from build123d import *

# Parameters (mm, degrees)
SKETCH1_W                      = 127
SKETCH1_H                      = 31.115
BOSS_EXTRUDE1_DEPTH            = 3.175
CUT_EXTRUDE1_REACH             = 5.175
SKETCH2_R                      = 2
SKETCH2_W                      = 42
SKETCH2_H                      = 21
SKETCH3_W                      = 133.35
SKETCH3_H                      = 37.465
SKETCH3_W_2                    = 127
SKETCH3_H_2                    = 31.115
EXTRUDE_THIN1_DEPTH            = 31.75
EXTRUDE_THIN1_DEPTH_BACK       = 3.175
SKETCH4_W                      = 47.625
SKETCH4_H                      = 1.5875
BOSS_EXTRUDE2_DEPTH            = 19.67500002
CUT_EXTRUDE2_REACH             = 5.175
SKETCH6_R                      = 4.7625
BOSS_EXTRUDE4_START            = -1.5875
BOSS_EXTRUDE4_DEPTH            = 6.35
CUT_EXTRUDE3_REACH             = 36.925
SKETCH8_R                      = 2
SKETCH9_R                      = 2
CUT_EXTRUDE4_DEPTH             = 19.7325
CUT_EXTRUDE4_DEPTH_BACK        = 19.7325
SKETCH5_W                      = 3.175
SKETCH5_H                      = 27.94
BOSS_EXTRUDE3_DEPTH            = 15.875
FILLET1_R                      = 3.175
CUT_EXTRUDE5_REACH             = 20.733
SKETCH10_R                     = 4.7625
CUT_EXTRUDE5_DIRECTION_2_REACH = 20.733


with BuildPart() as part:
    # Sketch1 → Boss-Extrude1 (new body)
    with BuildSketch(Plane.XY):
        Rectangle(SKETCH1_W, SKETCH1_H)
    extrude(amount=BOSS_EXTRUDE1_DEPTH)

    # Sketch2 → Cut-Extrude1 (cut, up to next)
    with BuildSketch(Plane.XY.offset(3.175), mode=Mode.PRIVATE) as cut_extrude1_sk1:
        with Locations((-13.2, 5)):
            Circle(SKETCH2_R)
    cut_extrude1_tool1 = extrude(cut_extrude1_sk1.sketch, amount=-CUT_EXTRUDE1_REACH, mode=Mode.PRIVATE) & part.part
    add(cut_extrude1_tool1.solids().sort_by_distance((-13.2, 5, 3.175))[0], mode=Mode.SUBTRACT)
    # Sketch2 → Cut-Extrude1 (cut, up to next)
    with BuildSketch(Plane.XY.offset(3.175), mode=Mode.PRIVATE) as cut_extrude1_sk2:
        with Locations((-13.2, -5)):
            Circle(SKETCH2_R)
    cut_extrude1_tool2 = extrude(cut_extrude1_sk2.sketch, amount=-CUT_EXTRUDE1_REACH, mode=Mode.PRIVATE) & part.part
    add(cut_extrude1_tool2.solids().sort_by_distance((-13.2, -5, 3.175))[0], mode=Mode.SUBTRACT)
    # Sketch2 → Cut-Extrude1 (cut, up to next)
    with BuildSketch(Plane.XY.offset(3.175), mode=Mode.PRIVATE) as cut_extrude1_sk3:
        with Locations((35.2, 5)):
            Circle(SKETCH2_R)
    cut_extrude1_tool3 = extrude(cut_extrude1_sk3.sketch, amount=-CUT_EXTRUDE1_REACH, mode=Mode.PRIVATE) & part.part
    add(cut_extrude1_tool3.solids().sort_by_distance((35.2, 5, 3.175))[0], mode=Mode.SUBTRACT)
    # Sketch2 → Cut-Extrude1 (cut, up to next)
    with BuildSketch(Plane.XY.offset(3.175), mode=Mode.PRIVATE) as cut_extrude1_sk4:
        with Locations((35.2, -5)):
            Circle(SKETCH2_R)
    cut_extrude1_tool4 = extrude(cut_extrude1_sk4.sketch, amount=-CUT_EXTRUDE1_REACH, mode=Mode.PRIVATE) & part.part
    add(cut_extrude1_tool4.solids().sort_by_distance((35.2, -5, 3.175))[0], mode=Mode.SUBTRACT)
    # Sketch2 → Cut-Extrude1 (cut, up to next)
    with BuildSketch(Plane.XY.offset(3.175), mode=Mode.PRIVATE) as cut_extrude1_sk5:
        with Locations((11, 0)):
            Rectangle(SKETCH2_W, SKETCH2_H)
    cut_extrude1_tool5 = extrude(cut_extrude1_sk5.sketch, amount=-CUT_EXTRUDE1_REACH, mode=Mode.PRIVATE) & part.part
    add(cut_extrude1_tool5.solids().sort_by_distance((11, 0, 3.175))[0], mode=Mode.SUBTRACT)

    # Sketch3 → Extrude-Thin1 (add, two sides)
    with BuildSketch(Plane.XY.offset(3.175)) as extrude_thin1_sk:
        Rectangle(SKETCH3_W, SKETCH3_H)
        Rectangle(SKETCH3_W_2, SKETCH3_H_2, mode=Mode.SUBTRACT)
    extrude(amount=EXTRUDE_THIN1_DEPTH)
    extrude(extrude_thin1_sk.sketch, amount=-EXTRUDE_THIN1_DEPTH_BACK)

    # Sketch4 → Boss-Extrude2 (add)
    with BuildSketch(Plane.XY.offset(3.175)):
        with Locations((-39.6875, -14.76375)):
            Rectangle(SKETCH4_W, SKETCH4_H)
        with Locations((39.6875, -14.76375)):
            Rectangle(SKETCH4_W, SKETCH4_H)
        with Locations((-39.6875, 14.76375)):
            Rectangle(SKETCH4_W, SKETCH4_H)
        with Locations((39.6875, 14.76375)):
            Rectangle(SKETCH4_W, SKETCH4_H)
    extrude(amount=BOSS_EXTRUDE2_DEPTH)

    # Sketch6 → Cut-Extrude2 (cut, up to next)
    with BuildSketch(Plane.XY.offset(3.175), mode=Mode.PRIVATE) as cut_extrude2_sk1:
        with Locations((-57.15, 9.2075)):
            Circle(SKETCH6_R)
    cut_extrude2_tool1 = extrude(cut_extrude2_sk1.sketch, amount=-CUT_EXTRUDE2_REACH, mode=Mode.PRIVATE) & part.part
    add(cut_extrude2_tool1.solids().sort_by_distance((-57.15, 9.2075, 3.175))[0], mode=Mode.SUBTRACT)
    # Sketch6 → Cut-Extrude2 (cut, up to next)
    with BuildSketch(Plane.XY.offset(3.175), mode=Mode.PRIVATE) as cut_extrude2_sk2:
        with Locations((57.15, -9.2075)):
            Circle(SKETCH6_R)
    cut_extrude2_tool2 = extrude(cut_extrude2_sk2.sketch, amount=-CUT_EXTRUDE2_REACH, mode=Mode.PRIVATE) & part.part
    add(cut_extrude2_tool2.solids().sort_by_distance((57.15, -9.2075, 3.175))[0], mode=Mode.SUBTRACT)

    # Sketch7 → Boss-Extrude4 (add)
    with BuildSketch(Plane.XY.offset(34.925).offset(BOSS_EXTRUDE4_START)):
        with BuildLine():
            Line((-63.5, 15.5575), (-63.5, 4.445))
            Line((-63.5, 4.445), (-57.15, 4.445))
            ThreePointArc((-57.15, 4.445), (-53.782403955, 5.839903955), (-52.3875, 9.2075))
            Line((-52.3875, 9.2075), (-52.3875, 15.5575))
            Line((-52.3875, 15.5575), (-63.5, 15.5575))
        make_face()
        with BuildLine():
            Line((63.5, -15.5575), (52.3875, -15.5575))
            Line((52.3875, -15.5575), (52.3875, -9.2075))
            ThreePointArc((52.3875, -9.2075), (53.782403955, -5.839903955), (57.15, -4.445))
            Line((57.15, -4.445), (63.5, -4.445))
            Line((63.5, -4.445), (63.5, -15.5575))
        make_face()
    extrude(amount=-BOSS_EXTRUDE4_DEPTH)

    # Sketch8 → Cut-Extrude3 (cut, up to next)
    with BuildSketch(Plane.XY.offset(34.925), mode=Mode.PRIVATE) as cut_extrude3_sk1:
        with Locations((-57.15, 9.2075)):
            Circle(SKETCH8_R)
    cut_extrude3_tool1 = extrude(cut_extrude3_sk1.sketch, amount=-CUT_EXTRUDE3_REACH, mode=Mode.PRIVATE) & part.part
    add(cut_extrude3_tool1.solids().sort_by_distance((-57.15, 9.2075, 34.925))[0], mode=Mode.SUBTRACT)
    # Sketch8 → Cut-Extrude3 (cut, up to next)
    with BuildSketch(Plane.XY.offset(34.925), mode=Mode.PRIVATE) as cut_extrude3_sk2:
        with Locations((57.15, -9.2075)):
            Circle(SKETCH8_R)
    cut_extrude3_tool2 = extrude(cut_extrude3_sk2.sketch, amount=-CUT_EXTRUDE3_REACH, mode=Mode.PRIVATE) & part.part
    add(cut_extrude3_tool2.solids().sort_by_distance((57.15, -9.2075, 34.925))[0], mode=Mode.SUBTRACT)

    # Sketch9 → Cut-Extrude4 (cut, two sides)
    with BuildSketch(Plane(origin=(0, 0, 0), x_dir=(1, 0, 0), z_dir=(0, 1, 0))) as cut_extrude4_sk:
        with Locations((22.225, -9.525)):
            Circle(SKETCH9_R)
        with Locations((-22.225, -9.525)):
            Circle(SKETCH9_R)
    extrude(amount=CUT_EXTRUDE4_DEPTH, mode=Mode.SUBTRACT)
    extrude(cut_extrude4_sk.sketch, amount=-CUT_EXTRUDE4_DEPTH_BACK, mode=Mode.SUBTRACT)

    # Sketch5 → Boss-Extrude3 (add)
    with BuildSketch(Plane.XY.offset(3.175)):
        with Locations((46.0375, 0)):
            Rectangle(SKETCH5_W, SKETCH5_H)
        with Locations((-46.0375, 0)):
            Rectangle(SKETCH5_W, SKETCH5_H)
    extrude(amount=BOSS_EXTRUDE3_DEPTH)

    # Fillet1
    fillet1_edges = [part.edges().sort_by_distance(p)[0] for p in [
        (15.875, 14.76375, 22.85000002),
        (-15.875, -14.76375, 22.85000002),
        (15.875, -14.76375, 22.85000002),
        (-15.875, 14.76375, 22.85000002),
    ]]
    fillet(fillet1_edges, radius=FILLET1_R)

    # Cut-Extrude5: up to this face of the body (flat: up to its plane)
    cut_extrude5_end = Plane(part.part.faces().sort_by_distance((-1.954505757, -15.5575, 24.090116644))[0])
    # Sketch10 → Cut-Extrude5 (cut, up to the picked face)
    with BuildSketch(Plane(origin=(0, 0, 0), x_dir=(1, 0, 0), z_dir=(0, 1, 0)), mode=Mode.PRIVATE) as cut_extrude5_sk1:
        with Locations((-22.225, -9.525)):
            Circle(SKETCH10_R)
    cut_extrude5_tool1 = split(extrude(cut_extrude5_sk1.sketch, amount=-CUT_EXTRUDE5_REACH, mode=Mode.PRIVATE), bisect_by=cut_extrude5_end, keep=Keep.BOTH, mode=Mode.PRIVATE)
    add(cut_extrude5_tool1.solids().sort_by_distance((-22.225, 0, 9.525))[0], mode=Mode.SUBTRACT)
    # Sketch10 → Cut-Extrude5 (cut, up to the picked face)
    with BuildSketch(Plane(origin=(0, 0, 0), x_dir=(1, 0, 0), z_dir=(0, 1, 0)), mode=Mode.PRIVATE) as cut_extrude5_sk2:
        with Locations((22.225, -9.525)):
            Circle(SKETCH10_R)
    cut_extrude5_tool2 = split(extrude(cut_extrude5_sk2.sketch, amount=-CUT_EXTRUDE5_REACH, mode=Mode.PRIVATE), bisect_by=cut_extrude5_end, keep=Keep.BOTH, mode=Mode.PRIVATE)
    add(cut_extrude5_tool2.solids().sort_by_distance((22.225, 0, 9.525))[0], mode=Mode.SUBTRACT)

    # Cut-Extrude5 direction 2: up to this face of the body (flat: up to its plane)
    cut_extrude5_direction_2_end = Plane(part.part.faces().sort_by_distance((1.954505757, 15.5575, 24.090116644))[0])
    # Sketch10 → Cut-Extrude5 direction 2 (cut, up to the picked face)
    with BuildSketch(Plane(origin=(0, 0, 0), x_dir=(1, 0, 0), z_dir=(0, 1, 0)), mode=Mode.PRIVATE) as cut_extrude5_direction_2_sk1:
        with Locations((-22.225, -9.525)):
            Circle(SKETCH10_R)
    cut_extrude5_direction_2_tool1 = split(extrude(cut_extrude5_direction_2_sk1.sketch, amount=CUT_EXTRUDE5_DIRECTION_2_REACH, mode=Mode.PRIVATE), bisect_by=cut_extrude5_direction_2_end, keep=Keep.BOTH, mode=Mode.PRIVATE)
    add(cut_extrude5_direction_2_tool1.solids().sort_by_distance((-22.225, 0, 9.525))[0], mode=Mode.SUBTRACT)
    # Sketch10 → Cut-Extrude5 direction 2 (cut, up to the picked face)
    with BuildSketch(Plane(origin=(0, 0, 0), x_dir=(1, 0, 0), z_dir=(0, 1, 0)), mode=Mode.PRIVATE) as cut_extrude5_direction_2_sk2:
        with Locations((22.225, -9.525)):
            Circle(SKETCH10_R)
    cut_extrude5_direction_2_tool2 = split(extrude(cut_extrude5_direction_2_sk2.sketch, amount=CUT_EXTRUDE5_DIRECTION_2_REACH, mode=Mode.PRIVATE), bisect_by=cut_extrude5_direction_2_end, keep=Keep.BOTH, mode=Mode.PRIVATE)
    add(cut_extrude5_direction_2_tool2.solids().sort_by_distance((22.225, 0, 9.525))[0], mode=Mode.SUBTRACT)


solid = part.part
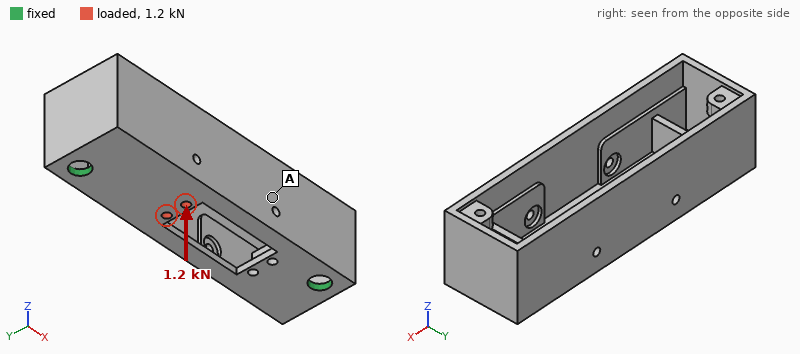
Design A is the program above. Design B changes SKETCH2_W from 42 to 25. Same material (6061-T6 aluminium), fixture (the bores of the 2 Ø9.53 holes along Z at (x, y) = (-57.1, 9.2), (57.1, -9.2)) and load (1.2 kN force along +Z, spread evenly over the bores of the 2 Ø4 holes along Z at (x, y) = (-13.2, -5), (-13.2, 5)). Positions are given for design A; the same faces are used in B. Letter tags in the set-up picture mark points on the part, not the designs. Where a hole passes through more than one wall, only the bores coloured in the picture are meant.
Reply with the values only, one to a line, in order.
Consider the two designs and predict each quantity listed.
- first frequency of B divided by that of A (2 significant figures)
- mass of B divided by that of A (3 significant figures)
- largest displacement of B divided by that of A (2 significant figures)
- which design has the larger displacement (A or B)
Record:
1.0
1.02
0.59
A
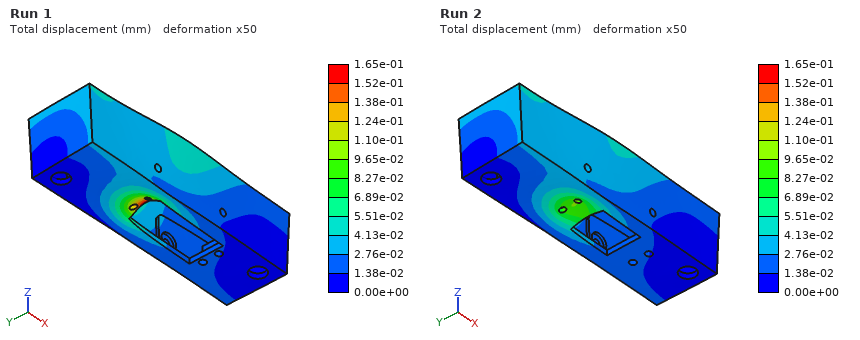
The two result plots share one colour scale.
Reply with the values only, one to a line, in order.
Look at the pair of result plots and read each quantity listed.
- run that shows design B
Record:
Run 2
